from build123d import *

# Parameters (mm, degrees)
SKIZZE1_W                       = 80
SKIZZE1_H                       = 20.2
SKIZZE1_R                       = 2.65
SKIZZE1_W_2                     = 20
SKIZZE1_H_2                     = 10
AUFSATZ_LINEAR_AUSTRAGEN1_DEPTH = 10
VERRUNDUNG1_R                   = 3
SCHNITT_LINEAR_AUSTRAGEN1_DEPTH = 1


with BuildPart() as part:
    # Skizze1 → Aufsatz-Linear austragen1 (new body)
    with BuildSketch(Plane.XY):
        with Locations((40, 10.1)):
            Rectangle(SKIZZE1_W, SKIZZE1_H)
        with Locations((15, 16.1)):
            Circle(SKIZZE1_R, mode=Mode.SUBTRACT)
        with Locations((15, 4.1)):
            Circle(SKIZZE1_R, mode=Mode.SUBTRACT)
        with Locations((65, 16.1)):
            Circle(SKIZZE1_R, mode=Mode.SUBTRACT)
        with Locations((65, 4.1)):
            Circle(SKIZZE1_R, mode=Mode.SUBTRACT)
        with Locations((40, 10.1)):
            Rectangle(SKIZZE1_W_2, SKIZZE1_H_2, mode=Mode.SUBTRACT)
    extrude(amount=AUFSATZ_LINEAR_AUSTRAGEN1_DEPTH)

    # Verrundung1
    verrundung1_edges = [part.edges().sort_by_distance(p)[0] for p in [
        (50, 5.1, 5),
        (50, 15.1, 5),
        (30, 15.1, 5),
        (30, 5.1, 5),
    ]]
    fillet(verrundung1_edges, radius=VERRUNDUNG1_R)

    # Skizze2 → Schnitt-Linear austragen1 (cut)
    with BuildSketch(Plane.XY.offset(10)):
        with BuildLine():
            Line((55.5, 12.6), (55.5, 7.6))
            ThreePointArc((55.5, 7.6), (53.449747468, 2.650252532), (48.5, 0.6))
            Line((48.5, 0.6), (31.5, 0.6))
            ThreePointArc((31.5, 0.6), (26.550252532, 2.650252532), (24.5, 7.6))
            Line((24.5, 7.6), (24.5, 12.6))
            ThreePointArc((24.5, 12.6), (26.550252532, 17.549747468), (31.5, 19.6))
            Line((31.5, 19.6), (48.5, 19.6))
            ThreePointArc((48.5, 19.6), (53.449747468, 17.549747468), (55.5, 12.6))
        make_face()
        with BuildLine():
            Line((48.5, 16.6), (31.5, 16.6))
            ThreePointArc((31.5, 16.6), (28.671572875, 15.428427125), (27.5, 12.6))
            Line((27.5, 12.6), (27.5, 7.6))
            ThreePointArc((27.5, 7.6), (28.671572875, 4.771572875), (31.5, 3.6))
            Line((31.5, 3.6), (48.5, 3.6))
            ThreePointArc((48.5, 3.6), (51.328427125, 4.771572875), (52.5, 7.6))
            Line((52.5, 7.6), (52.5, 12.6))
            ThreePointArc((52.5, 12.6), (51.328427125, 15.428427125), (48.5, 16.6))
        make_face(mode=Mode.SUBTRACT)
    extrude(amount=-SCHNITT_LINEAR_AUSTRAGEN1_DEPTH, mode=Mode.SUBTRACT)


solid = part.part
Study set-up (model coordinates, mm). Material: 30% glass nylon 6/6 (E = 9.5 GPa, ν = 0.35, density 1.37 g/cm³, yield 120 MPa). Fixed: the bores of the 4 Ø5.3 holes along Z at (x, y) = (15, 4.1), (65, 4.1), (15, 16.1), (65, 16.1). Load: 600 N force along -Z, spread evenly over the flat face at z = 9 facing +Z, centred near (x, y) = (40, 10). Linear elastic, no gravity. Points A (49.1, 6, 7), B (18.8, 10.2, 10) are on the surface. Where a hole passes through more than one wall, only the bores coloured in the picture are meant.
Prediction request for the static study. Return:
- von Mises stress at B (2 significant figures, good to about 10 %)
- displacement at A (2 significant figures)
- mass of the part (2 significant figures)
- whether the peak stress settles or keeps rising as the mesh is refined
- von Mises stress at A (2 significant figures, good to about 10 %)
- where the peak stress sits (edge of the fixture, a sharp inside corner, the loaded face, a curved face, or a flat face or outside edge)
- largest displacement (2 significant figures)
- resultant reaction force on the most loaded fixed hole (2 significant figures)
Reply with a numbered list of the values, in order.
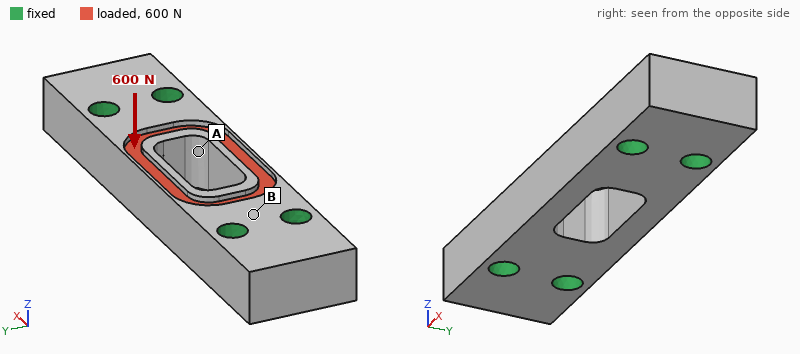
1. 4.5 MPa
2. 18 µm
3. 18 g
4. keeps rising
5. 1.8 MPa
6. edge of the fixture
7. 28 µm
8. 150 N
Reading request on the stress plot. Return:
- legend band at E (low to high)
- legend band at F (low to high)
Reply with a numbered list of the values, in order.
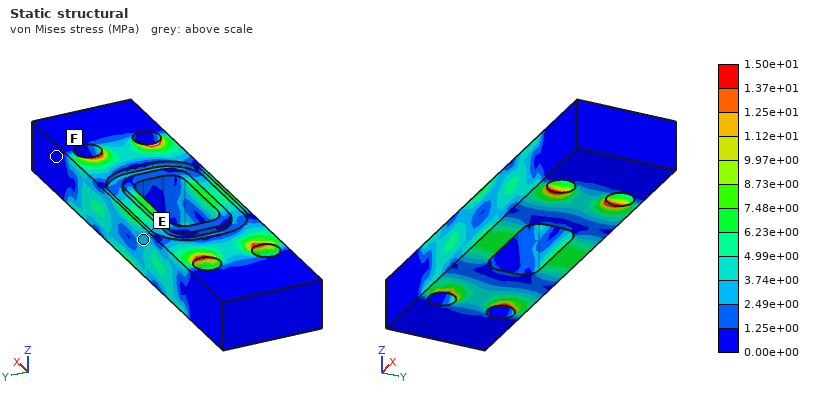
1. 2.49e+00 to 3.74e+00 MPa
2. 0.00e+00 to 1.25e+00 MPa
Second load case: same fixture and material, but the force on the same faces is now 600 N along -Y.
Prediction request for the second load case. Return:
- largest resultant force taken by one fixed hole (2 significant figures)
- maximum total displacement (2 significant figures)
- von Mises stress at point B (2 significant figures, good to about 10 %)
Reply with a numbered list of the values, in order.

1. 250 N
2. 36 µm
3. 5.2 MPa
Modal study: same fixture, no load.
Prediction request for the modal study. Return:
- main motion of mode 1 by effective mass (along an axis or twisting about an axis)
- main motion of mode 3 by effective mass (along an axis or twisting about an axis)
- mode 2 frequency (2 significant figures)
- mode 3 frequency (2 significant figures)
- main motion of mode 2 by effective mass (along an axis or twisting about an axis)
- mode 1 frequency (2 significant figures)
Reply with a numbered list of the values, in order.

1. along Z
2. along Y
3. 14 kHz
4. 15 kHz
5. twisting about X
6. 11 kHz
